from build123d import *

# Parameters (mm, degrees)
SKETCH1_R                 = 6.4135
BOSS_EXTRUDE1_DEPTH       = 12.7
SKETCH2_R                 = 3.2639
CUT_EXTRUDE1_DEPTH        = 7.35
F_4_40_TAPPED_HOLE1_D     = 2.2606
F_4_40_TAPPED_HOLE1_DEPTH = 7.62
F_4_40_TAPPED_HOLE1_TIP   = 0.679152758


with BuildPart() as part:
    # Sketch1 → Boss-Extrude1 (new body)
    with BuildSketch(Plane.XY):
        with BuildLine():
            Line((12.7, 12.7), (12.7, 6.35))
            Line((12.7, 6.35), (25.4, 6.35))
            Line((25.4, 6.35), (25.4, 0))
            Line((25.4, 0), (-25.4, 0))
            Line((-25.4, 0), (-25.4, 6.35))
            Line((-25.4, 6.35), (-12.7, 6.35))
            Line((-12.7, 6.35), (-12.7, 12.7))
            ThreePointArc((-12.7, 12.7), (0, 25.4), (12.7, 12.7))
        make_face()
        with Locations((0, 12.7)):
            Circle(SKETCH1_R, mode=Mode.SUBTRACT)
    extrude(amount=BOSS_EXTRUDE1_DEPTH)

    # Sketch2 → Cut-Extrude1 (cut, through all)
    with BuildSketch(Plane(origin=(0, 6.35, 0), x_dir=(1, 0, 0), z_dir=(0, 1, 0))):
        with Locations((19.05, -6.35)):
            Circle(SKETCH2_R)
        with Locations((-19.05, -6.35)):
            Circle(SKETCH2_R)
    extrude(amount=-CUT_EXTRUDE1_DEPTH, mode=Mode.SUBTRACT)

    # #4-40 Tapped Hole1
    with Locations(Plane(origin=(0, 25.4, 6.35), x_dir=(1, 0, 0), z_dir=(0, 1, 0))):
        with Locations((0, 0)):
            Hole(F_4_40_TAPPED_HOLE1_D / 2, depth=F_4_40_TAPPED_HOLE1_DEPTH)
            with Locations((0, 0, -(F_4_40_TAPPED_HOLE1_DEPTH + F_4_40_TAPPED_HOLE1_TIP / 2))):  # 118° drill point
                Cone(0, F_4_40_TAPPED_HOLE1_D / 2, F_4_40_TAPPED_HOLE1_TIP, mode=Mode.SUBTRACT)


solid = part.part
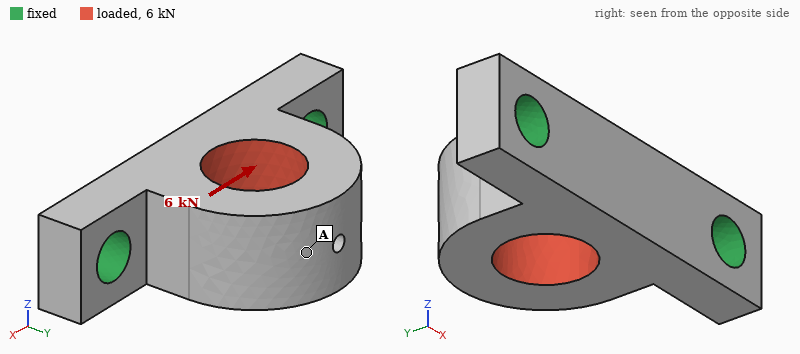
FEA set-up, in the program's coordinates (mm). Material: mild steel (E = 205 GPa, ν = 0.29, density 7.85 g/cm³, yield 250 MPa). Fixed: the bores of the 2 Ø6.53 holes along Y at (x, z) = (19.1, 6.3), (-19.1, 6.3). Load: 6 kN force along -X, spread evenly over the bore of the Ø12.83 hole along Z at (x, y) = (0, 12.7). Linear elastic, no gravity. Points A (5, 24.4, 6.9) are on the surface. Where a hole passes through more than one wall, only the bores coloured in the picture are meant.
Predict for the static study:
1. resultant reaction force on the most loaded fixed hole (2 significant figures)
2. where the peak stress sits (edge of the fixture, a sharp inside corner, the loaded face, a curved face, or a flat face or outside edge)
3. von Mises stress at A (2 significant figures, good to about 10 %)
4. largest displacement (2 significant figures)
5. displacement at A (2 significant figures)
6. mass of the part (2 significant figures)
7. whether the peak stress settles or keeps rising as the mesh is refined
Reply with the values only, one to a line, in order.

3.5 kN
edge of the fixture
23 MPa
13 µm
13 µm
57 g
keeps rising
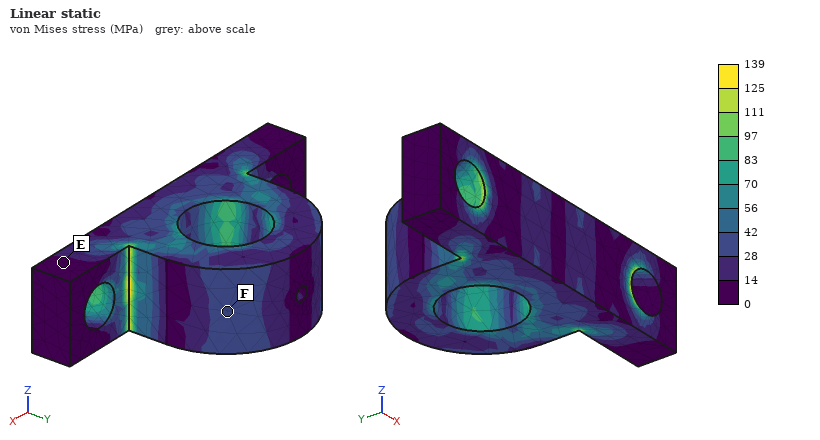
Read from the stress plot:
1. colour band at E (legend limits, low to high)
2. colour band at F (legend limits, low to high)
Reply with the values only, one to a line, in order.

0 to 14 MPa
28 to 42 MPa
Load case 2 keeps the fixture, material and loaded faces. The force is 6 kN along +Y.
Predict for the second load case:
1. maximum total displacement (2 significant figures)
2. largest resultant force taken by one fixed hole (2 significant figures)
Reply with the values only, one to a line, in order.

9.7 µm
3.1 kN
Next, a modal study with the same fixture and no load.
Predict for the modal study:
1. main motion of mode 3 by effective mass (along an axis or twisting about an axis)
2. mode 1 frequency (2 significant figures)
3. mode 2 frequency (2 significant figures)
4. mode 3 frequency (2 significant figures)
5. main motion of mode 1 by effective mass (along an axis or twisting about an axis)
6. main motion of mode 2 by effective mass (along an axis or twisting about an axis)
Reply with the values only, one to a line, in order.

along Y
8800 Hz
19 kHz
22 kHz
along Z
along X
